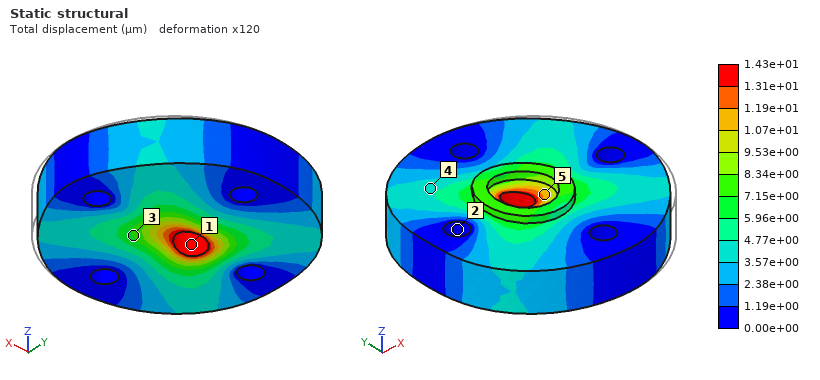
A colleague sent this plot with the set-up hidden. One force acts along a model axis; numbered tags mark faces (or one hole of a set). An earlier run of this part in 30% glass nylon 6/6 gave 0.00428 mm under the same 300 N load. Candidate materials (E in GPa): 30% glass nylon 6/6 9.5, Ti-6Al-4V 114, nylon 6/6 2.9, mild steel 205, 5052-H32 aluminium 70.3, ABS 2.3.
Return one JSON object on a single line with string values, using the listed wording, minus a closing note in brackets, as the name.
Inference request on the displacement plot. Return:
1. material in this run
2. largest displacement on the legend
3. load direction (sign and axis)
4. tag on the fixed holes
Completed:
{"material in this run": "nylon 6/6", "largest displacement on the legend": "1.43e+01 µm", "load direction": "-X", "tag on the fixed holes": "2"}
